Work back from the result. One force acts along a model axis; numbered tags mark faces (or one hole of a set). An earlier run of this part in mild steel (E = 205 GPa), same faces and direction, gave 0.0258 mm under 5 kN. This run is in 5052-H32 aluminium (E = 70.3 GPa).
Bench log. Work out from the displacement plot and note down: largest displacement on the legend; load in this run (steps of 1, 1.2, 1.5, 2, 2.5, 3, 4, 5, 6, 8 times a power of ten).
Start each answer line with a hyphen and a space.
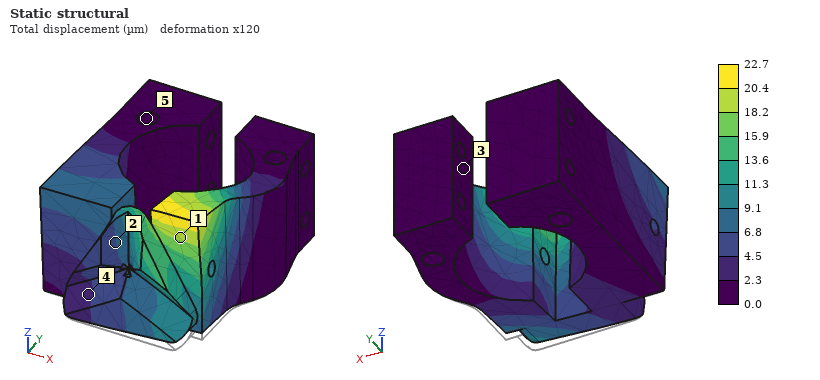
- 22.7 µm
- 1.5 kN
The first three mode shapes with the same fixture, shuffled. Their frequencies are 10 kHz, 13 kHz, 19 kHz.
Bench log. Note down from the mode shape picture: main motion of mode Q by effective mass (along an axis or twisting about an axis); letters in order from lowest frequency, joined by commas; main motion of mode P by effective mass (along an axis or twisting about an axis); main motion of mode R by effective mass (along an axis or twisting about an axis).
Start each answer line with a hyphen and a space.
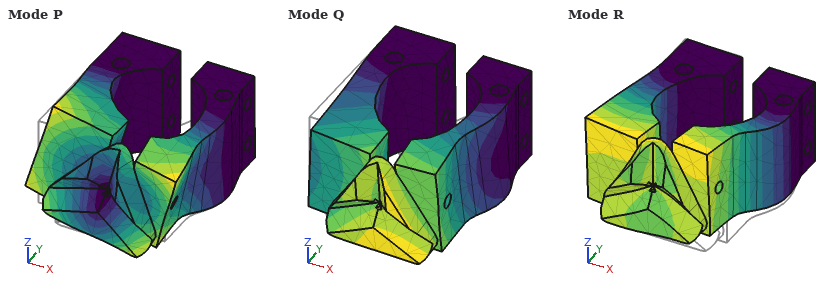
- along Z
- R, Q, P
- twisting about Y
- along X
